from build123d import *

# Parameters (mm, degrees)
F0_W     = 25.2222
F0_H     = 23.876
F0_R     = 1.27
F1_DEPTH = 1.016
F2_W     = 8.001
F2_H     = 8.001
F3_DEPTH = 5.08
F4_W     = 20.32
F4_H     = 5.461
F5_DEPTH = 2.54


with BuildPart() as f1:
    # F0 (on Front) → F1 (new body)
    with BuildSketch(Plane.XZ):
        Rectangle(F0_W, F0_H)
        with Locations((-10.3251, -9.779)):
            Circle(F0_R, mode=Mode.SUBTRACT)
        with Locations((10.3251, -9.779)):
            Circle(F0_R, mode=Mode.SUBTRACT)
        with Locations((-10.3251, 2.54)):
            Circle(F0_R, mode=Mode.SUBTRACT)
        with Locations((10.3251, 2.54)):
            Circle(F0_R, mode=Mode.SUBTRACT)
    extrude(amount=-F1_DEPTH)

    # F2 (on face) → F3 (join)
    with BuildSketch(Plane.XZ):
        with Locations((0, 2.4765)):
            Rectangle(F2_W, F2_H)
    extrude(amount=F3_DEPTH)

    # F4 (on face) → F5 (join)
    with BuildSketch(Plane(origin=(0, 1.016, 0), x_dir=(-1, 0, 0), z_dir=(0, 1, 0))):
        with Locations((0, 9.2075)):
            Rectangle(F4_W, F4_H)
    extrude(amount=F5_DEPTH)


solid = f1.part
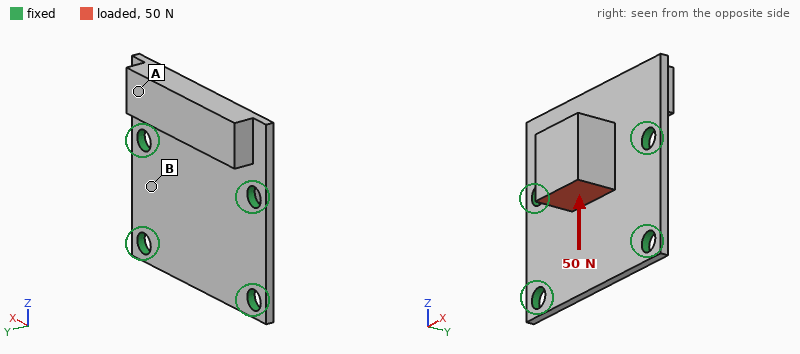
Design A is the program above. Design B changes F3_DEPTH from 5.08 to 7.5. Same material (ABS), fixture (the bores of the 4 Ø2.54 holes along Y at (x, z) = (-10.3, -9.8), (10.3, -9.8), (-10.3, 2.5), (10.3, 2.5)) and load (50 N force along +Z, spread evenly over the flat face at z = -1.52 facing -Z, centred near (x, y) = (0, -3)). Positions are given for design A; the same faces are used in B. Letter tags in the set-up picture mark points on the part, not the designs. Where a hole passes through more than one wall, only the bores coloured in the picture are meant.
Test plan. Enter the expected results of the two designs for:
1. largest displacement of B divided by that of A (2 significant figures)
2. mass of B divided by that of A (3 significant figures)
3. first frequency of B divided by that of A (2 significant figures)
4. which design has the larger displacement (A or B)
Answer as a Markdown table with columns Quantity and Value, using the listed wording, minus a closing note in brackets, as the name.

| Quantity | Value |
|---|---|
| largest displacement of B divided by that of A | 1.5 |
| mass of B divided by that of A | 1.13 |
| first frequency of B divided by that of A | 0.93 |
| which design has the larger displacement | B |
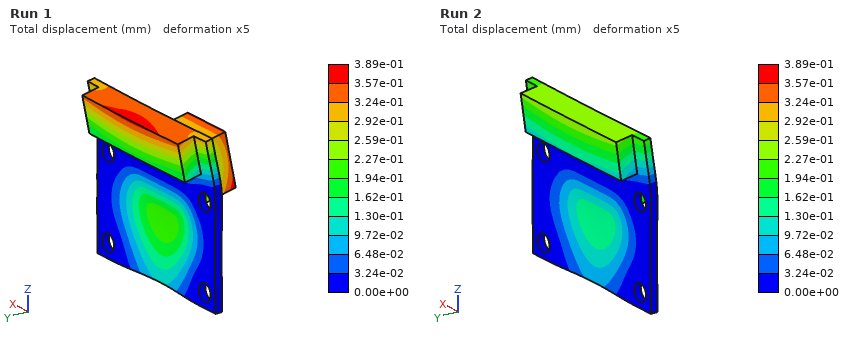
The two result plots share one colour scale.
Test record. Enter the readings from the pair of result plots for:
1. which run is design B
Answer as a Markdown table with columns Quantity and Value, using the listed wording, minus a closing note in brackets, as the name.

| Quantity | Value |
|---|---|
| which run is design B | Run 1 |
